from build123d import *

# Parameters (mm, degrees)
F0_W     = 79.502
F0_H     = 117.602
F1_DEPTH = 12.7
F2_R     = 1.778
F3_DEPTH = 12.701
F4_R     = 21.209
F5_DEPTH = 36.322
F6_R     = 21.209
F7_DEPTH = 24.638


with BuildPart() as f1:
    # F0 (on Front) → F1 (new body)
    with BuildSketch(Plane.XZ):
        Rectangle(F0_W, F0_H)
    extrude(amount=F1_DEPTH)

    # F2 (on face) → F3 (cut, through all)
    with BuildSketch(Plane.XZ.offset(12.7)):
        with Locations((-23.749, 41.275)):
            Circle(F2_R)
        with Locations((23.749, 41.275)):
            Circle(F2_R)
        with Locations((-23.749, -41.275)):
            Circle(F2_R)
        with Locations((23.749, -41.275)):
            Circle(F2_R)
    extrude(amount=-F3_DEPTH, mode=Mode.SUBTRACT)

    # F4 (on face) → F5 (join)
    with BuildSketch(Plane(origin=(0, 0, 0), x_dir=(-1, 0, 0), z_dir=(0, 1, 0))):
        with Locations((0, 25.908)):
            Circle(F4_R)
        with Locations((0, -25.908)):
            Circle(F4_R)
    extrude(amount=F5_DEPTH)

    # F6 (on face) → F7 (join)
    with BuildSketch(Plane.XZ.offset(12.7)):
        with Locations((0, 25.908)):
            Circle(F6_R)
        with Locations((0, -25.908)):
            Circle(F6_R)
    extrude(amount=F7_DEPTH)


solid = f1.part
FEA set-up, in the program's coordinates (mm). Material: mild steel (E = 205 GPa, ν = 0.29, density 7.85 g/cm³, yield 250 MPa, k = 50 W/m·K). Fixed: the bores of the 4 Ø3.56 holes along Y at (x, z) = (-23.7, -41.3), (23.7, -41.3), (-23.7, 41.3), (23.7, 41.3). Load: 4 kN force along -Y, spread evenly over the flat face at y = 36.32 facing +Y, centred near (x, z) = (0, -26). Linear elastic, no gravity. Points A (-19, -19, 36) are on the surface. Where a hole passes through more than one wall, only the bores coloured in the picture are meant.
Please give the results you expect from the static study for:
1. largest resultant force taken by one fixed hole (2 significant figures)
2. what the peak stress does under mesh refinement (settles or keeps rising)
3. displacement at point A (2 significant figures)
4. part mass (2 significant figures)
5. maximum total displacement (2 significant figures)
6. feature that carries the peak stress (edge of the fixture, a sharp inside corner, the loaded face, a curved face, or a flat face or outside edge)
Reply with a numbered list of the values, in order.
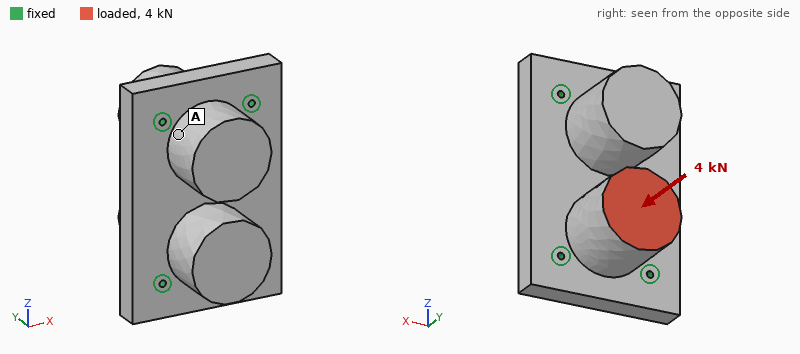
1. 1.6 kN
2. keeps rising
3. 1.1 µm
4. 2.3 kg
5. 4.9 µm
6. edge of the fixture
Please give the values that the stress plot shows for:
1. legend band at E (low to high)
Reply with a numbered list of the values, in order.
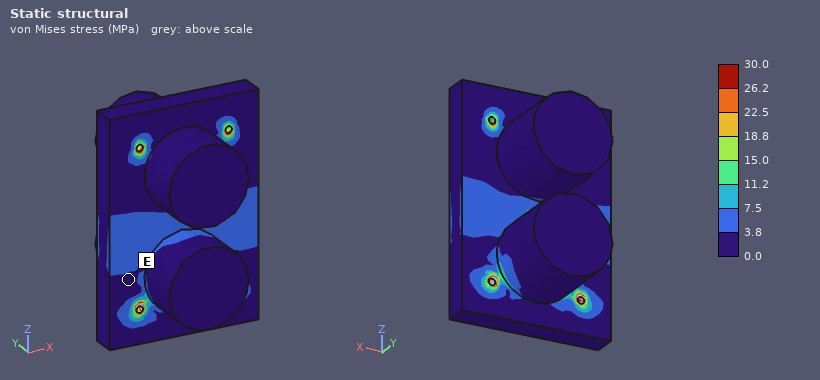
1. 0.0 to 3.8 MPa
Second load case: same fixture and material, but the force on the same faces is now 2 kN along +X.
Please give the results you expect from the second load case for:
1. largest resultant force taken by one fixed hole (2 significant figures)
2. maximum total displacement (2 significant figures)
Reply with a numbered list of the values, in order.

1. 1.8 kN
2. 5.0 µm
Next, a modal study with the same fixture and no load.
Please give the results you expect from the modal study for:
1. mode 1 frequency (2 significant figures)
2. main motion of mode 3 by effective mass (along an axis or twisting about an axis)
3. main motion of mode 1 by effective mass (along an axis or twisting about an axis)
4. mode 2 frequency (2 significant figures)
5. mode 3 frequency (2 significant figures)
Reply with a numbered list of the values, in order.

1. 3500 Hz
2. along Z
3. along Y
4. 6700 Hz
5. 8200 Hz
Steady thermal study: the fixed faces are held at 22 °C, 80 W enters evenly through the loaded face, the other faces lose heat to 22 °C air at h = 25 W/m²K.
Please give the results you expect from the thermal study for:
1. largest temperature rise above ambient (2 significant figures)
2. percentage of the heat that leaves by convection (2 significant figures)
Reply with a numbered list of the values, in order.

1. 64 K
2. 16 %
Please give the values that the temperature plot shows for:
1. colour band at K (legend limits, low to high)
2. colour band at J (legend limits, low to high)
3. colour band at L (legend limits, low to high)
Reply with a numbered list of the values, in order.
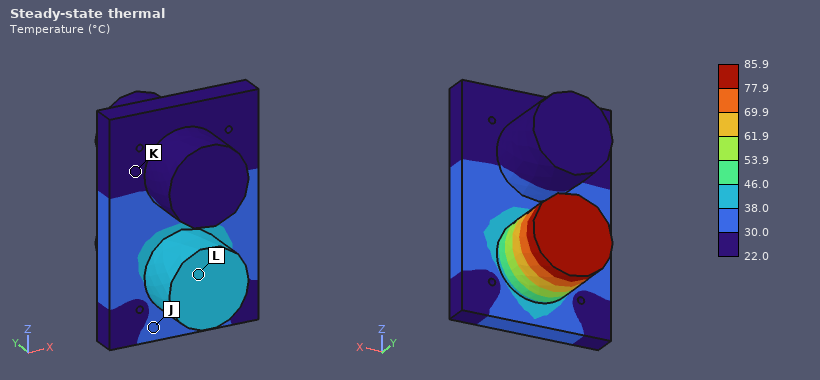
1. 22.0 to 30.0 °C
2. 30.0 to 38.0 °C
3. 38.0 to 46.0 °C
